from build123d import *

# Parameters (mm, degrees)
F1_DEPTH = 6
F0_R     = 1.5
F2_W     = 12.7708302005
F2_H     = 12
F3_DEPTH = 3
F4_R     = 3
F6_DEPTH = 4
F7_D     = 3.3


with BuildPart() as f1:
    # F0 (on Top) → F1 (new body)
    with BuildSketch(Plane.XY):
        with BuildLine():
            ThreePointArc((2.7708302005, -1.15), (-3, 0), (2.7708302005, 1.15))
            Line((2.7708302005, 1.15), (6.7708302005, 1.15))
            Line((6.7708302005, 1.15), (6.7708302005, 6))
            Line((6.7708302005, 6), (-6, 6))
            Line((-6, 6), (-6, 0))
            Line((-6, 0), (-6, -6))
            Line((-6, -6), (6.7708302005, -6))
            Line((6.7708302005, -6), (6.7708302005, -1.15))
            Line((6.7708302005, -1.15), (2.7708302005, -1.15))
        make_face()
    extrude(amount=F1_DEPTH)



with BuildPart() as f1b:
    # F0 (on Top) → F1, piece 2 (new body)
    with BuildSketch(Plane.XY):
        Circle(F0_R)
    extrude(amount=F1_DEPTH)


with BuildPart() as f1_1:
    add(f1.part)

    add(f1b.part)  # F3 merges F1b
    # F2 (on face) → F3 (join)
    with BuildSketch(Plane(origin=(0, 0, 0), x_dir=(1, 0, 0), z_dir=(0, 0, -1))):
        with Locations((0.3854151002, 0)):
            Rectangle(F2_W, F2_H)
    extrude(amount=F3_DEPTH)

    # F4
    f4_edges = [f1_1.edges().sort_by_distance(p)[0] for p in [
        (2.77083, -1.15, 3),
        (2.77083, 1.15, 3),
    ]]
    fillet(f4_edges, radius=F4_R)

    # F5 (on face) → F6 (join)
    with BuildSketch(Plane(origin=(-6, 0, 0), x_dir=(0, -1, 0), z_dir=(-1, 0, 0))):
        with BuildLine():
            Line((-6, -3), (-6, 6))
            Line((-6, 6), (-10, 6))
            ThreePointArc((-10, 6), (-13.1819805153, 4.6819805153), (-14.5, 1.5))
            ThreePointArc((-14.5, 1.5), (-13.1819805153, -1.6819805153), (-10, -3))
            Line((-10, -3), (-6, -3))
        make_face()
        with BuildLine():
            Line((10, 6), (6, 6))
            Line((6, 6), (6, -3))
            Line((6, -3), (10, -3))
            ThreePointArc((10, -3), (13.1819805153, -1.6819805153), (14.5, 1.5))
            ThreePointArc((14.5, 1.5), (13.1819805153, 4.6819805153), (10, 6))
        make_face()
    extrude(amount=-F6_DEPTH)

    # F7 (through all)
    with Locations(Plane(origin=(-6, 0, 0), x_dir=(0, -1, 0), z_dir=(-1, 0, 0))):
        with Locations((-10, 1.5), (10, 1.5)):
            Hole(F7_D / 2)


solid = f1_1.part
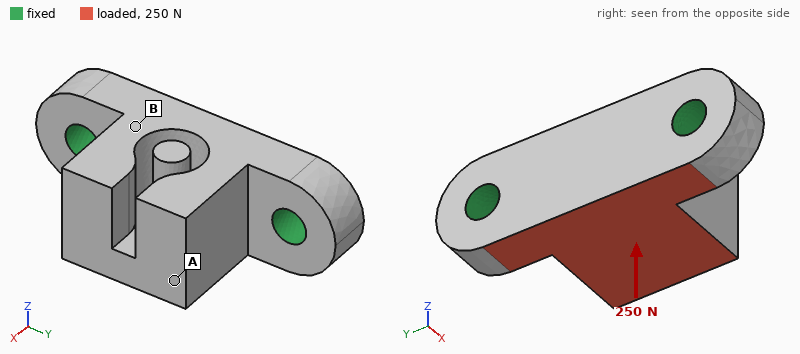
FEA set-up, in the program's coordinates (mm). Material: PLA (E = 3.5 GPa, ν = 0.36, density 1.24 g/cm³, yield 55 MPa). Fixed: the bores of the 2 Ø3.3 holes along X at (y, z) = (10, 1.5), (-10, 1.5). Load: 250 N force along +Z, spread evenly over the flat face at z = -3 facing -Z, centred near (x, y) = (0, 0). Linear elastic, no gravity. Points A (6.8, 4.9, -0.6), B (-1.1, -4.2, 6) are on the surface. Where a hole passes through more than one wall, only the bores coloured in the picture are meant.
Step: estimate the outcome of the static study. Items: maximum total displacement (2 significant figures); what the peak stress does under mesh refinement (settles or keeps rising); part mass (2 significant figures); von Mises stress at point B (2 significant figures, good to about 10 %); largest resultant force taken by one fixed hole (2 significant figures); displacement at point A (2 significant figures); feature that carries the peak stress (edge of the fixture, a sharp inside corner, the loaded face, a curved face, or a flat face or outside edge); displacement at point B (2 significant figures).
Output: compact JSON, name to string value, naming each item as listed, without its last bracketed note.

{"maximum total displacement": "0.15 mm", "what the peak stress does under mesh refinement": "keeps rising", "part mass": "2.1 g", "von Mises stress at point B": "4.9 MPa", "largest resultant force taken by one fixed hole": "130 N", "displacement at point A": "0.14 mm", "feature that carries the peak stress": "edge of the fixture", "displacement at point B": "0.064 mm"}
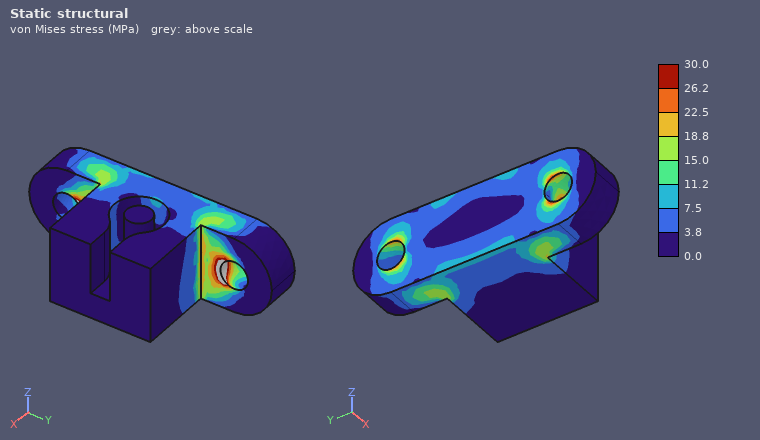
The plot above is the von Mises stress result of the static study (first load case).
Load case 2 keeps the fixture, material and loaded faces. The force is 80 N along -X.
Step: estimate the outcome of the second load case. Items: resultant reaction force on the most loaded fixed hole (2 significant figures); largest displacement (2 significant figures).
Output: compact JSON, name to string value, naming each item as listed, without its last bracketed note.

{"resultant reaction force on the most loaded fixed hole": "41 N", "largest displacement": "48 µm"}
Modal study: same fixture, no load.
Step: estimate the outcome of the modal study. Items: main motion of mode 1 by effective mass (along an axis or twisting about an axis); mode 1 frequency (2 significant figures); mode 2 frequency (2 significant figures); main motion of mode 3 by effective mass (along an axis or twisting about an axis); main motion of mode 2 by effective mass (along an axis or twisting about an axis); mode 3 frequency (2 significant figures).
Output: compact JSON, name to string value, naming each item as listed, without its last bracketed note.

{"main motion of mode 1 by effective mass": "along Z", "mode 1 frequency": "5900 Hz", "mode 2 frequency": "10 kHz", "main motion of mode 3 by effective mass": "along X", "main motion of mode 2 by effective mass": "along Y", "mode 3 frequency": "11 kHz"}
